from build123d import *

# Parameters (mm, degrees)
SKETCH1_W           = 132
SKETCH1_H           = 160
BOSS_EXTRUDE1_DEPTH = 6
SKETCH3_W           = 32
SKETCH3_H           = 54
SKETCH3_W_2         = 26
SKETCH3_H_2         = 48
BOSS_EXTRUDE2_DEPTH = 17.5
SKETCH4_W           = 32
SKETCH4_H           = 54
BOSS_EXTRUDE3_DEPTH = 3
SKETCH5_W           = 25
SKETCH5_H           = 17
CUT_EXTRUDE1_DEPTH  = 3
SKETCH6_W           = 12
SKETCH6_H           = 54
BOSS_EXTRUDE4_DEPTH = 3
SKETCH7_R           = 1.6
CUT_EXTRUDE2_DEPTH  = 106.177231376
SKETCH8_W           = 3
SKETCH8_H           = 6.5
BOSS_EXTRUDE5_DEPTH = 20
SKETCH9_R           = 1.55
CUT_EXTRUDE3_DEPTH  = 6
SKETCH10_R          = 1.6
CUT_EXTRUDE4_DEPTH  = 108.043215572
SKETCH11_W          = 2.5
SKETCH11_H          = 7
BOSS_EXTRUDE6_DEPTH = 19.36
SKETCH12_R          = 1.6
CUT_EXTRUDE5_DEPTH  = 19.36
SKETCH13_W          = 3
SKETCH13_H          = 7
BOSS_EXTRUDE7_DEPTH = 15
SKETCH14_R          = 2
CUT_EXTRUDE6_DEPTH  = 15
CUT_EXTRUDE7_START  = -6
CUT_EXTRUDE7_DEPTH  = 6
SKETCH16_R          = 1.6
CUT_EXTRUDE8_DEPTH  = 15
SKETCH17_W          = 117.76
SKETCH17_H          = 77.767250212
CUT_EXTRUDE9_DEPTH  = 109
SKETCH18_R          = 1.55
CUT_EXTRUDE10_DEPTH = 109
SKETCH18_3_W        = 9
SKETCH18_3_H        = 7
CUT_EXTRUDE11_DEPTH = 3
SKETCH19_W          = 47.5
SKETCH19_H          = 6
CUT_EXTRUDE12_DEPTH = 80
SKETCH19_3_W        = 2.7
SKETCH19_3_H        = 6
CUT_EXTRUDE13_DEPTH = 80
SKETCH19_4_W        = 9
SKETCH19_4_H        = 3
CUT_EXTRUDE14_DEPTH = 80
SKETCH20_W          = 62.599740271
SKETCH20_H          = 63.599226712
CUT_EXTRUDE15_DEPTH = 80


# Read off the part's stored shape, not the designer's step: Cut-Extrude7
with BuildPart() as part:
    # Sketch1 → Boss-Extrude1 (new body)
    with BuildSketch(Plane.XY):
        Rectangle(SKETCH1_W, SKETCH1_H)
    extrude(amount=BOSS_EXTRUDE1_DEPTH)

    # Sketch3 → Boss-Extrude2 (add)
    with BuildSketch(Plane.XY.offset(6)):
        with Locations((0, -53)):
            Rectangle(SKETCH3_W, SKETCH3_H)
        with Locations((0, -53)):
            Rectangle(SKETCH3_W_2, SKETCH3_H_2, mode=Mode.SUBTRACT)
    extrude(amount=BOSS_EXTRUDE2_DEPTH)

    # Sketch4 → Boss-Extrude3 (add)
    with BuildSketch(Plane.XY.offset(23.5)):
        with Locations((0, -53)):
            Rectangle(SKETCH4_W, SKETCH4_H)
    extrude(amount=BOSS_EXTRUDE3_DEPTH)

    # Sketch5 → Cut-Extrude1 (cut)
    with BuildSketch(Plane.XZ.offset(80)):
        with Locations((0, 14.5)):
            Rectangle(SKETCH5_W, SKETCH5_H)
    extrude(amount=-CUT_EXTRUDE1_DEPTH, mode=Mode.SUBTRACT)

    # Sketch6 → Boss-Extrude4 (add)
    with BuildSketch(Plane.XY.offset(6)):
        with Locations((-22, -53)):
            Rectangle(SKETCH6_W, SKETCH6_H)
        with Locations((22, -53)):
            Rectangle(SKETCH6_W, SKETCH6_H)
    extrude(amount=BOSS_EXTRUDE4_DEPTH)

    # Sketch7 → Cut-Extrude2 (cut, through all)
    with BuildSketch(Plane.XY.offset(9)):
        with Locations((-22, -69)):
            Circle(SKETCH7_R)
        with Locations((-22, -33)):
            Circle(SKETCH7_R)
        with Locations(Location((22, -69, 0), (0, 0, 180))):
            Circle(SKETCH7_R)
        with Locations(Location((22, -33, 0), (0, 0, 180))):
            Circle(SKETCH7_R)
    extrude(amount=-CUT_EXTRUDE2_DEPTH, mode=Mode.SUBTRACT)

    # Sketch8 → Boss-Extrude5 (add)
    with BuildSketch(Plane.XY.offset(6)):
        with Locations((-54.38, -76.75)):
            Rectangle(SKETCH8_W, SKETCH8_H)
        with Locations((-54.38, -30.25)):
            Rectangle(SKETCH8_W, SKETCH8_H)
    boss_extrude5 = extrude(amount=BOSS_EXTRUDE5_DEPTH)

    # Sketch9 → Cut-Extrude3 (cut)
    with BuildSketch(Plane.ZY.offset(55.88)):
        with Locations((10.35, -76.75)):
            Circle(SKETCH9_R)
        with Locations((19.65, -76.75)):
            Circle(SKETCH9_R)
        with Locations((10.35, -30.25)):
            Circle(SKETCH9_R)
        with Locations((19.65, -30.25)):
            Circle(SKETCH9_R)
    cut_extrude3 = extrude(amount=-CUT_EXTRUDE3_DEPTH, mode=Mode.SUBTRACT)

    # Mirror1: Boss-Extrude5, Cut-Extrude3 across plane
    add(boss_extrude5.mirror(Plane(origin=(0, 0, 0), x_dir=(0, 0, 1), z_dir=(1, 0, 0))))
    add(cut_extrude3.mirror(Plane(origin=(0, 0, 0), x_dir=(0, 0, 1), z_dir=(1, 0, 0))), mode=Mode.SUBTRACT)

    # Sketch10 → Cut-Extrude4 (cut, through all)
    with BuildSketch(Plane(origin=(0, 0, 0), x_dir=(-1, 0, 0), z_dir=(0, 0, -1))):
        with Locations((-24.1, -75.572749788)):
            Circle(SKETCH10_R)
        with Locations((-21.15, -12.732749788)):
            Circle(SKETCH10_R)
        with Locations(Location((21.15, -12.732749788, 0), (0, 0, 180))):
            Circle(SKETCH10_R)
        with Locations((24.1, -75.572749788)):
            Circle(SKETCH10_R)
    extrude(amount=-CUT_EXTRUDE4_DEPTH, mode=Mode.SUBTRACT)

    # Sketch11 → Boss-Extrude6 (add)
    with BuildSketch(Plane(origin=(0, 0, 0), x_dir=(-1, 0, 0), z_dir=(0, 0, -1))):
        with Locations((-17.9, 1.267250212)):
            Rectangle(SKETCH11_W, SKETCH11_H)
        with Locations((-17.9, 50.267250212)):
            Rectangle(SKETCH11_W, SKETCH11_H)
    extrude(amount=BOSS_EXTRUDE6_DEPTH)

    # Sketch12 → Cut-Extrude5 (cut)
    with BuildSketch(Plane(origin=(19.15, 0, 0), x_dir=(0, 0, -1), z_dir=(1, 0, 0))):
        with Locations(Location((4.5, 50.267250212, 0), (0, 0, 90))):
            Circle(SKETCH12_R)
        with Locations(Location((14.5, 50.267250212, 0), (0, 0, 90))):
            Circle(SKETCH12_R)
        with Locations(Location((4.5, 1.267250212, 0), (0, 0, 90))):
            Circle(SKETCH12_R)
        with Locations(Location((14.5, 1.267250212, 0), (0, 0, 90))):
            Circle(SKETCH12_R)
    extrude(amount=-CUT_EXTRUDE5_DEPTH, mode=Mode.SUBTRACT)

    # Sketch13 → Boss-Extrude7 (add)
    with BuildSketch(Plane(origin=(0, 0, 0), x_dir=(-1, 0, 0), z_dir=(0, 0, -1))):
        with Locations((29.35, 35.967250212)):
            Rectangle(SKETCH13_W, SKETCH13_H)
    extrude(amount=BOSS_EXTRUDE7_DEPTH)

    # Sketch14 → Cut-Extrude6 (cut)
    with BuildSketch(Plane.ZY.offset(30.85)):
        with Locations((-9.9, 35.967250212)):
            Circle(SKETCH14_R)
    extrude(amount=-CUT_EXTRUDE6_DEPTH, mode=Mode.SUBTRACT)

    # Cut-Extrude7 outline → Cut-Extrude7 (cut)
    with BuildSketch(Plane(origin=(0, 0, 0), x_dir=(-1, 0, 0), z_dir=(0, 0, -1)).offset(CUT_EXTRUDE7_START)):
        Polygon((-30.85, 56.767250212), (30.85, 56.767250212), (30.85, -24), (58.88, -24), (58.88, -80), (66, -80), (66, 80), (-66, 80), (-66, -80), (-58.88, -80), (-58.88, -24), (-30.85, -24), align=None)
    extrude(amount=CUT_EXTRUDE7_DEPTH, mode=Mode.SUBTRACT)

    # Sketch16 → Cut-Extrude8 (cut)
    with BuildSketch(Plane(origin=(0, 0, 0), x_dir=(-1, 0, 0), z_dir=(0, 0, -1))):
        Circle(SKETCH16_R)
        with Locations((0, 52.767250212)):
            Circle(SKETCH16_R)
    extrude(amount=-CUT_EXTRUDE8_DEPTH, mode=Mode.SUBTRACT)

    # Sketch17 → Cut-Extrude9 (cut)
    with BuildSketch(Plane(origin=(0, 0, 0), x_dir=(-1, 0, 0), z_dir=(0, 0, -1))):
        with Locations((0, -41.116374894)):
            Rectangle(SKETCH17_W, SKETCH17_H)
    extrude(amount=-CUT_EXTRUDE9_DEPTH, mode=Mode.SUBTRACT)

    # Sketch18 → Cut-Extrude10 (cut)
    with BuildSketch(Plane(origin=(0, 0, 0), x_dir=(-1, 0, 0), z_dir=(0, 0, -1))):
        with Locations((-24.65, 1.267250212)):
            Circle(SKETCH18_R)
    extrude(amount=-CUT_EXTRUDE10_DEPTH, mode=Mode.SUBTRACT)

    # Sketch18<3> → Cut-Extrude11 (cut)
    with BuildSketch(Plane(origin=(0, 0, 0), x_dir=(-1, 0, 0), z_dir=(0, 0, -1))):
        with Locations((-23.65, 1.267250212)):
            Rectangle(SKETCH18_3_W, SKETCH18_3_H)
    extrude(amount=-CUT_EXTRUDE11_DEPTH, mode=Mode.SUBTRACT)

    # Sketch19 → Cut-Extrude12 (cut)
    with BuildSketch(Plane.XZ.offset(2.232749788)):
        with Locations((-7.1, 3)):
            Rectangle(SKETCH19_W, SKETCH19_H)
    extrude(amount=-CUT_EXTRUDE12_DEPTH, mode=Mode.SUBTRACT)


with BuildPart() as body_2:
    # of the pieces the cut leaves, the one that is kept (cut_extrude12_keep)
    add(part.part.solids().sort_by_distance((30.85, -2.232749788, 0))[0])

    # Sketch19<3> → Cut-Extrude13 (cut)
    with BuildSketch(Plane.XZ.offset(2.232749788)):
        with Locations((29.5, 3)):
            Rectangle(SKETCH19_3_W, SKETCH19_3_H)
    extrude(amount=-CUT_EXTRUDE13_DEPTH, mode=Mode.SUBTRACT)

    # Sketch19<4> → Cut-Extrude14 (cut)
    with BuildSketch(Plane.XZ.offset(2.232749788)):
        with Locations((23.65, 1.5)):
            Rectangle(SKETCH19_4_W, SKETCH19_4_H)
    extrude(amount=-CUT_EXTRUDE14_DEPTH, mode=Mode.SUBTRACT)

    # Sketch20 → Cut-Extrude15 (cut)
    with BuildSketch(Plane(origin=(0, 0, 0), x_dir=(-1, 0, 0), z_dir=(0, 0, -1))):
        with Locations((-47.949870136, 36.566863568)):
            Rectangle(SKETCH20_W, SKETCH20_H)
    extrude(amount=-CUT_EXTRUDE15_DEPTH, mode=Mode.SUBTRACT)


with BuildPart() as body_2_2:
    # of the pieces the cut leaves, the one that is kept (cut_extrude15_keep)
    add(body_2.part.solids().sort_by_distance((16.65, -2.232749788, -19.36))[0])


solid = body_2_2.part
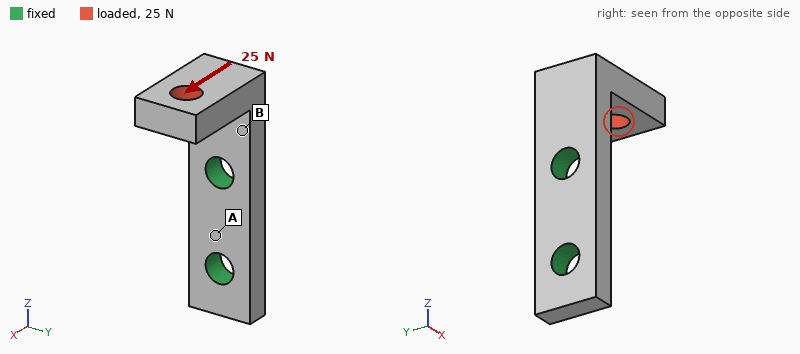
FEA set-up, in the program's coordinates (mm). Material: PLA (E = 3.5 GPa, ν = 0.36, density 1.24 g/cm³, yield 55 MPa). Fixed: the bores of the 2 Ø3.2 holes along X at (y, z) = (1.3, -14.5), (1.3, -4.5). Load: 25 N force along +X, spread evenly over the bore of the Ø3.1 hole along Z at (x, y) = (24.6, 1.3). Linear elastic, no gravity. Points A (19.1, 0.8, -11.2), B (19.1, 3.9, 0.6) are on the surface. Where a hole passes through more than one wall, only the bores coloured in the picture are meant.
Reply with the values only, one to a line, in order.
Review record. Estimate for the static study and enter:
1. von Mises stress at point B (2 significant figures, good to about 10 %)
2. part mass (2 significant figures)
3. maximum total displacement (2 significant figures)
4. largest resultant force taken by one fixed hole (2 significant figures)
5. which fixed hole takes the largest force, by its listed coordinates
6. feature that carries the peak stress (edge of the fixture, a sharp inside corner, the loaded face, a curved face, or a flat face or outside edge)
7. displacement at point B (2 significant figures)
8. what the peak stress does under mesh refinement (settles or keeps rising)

13 MPa
0.71 g
0.31 mm
26 N
(1.3, -4.5)
edge of the fixture
0.052 mm
keeps rising
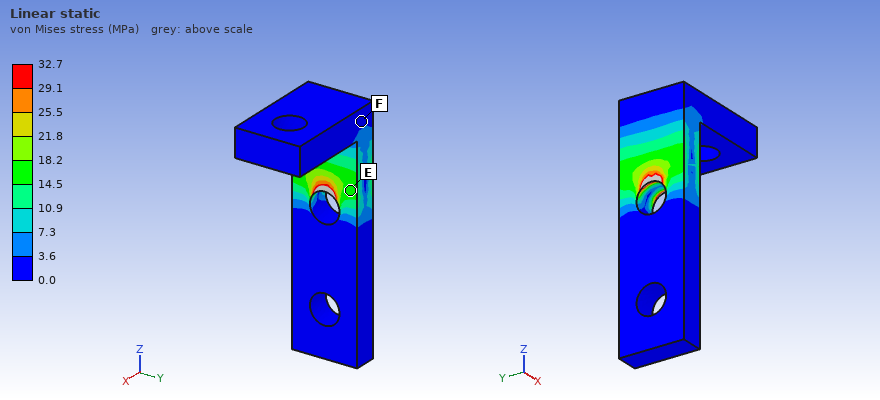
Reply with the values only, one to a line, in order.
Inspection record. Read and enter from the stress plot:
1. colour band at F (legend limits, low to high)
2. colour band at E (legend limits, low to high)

0.0 to 3.6 MPa
14.5 to 18.2 MPa
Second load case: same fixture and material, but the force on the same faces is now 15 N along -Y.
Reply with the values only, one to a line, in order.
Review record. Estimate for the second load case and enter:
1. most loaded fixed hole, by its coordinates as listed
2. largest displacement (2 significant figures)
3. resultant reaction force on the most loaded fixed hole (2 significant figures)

(1.3, -4.5)
0.21 mm
18 N
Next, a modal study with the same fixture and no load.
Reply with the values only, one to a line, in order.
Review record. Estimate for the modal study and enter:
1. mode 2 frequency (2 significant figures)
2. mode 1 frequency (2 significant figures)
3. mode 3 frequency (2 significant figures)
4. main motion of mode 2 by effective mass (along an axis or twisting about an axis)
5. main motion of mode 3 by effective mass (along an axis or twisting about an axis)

3700 Hz
2700 Hz
8100 Hz
along Y
along X
